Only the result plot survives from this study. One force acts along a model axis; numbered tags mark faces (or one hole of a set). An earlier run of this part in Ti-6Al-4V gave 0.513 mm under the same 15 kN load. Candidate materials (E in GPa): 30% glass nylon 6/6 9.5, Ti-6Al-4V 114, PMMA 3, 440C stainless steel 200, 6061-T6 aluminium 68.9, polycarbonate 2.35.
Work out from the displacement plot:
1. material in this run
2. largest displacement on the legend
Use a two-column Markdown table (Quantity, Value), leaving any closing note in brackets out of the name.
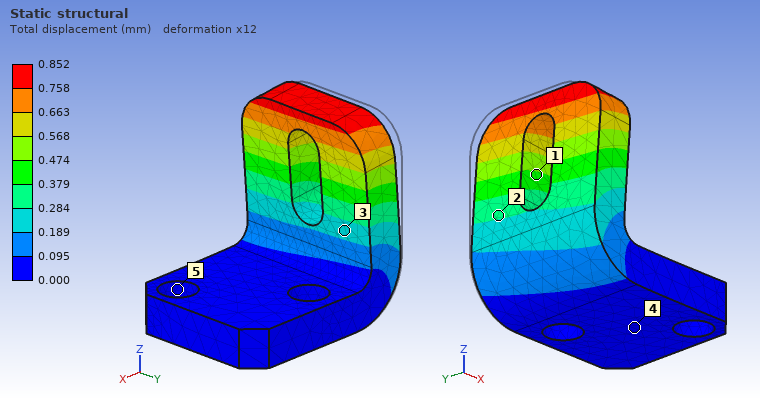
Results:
| Quantity | Value |
|---|---|
| material in this run | 6061-T6 aluminium |
| largest displacement on the legend | 0.852 mm |
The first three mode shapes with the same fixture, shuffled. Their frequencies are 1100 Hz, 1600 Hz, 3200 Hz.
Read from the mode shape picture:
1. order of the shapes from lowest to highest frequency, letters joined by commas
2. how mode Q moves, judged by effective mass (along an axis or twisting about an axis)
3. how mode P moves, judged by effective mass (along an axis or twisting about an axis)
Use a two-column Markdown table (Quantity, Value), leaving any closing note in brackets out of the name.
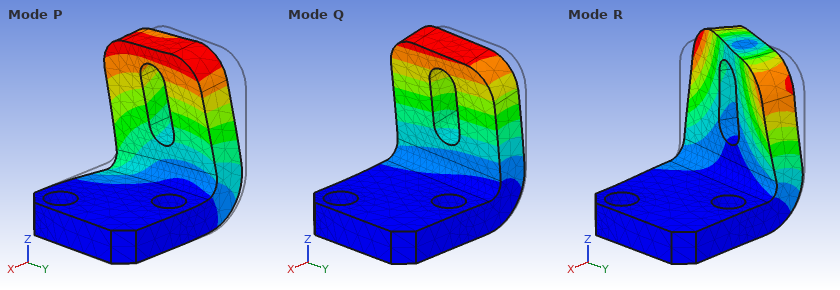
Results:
| Quantity | Value |
|---|---|
| order of the shapes from lowest to highest frequency, letters joined by commas | Q, P, R |
| how mode Q moves, judged by effective mass | along X |
| how mode P moves, judged by effective mass | along Y |
